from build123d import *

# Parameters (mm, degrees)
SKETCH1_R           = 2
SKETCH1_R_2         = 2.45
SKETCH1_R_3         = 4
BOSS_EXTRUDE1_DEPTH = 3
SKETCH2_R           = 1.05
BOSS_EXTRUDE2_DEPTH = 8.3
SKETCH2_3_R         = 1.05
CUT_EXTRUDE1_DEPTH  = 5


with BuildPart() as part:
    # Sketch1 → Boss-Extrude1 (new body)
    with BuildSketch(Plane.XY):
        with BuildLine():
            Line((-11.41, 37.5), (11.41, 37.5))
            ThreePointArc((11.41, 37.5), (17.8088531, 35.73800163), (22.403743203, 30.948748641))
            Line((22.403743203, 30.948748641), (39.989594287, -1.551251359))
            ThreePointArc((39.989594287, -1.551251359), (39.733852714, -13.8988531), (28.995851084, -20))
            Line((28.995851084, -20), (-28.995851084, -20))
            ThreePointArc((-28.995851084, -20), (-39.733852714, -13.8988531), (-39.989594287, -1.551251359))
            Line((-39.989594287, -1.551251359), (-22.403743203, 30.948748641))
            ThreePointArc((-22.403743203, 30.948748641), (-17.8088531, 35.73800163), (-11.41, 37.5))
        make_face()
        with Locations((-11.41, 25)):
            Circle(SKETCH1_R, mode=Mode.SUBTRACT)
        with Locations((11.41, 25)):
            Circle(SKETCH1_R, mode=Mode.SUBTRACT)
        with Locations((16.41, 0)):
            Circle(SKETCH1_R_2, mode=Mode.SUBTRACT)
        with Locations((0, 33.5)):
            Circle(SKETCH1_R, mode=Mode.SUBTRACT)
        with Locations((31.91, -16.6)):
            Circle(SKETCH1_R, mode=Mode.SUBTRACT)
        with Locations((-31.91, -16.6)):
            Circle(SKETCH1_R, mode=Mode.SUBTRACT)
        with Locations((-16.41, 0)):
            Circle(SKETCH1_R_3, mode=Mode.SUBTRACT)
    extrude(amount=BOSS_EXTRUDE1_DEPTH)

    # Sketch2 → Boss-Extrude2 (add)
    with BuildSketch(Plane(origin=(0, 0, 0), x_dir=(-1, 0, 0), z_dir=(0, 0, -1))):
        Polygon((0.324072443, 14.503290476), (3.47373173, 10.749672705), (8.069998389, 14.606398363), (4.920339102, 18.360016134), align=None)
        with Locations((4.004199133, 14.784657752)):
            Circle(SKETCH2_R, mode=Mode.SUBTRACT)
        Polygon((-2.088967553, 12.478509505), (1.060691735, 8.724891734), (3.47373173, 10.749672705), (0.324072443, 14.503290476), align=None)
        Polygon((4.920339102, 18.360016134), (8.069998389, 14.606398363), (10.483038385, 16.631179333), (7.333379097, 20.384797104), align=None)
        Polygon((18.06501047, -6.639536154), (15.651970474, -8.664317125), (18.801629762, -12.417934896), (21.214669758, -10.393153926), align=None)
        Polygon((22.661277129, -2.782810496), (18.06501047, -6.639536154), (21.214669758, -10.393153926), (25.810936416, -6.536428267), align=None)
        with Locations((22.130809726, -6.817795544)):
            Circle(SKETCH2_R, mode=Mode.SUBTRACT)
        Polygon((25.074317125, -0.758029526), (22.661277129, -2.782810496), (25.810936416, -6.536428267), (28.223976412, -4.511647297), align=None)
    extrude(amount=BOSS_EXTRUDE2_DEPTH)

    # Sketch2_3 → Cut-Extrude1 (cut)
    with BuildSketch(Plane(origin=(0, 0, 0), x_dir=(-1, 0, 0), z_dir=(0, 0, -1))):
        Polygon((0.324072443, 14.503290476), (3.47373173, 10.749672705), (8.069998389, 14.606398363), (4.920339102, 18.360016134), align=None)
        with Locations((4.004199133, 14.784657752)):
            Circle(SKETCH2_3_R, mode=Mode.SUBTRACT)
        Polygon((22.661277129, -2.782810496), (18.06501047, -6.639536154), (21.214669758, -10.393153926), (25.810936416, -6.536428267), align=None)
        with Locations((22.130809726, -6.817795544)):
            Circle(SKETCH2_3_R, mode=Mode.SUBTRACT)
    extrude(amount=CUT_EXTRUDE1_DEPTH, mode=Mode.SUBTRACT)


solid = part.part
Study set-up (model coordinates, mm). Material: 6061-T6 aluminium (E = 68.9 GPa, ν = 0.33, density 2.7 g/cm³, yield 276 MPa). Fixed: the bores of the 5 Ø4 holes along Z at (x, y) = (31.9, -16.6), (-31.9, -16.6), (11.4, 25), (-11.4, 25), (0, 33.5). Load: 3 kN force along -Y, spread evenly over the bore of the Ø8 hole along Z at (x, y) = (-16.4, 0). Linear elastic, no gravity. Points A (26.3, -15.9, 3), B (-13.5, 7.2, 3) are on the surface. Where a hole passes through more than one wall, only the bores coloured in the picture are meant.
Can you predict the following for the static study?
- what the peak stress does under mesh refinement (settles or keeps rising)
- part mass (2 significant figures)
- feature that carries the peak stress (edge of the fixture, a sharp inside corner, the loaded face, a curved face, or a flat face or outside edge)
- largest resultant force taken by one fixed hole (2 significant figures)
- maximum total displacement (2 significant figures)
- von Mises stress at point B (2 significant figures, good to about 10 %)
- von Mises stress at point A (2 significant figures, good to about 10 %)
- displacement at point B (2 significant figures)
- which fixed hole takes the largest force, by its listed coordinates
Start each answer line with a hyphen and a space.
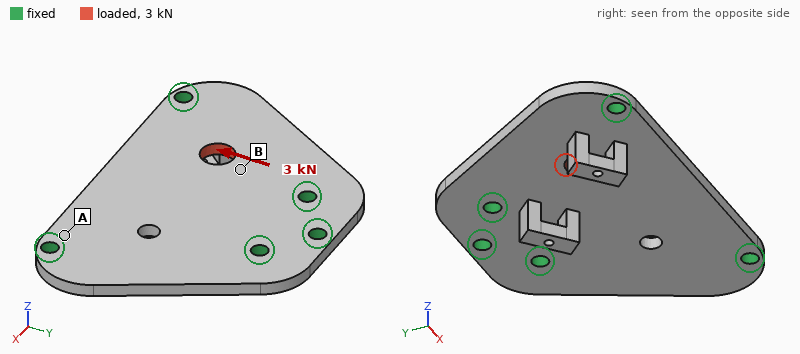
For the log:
- keeps rising
- 31 g
- edge of the fixture
- 1.2 kN
- 14 µm
- 40 MPa
- 11 MPa
- 8.8 µm
- (-11.4, 25)
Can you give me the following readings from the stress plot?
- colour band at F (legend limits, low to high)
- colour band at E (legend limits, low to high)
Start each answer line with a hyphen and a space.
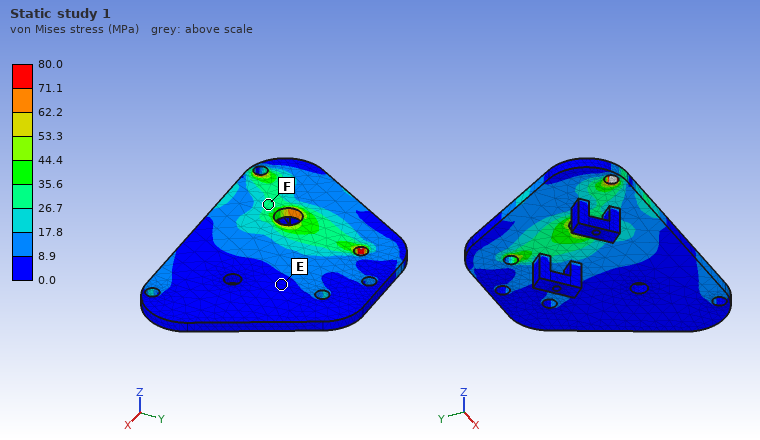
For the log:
- 26.7 to 35.6 MPa
- 0.0 to 8.9 MPa
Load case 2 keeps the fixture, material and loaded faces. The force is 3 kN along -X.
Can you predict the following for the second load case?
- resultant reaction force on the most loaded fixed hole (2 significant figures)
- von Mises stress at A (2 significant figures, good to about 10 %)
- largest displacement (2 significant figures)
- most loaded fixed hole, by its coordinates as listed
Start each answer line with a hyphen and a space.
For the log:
- 1.1 kN
- 24 MPa
- 15 µm
- (-31.9, -16.6)
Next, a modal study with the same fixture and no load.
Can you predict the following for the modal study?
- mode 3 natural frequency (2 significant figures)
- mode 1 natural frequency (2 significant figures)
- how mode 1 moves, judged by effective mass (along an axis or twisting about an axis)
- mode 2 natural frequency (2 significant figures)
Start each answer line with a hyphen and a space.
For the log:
- 6600 Hz
- 4200 Hz
- along Z
- 6400 Hz
